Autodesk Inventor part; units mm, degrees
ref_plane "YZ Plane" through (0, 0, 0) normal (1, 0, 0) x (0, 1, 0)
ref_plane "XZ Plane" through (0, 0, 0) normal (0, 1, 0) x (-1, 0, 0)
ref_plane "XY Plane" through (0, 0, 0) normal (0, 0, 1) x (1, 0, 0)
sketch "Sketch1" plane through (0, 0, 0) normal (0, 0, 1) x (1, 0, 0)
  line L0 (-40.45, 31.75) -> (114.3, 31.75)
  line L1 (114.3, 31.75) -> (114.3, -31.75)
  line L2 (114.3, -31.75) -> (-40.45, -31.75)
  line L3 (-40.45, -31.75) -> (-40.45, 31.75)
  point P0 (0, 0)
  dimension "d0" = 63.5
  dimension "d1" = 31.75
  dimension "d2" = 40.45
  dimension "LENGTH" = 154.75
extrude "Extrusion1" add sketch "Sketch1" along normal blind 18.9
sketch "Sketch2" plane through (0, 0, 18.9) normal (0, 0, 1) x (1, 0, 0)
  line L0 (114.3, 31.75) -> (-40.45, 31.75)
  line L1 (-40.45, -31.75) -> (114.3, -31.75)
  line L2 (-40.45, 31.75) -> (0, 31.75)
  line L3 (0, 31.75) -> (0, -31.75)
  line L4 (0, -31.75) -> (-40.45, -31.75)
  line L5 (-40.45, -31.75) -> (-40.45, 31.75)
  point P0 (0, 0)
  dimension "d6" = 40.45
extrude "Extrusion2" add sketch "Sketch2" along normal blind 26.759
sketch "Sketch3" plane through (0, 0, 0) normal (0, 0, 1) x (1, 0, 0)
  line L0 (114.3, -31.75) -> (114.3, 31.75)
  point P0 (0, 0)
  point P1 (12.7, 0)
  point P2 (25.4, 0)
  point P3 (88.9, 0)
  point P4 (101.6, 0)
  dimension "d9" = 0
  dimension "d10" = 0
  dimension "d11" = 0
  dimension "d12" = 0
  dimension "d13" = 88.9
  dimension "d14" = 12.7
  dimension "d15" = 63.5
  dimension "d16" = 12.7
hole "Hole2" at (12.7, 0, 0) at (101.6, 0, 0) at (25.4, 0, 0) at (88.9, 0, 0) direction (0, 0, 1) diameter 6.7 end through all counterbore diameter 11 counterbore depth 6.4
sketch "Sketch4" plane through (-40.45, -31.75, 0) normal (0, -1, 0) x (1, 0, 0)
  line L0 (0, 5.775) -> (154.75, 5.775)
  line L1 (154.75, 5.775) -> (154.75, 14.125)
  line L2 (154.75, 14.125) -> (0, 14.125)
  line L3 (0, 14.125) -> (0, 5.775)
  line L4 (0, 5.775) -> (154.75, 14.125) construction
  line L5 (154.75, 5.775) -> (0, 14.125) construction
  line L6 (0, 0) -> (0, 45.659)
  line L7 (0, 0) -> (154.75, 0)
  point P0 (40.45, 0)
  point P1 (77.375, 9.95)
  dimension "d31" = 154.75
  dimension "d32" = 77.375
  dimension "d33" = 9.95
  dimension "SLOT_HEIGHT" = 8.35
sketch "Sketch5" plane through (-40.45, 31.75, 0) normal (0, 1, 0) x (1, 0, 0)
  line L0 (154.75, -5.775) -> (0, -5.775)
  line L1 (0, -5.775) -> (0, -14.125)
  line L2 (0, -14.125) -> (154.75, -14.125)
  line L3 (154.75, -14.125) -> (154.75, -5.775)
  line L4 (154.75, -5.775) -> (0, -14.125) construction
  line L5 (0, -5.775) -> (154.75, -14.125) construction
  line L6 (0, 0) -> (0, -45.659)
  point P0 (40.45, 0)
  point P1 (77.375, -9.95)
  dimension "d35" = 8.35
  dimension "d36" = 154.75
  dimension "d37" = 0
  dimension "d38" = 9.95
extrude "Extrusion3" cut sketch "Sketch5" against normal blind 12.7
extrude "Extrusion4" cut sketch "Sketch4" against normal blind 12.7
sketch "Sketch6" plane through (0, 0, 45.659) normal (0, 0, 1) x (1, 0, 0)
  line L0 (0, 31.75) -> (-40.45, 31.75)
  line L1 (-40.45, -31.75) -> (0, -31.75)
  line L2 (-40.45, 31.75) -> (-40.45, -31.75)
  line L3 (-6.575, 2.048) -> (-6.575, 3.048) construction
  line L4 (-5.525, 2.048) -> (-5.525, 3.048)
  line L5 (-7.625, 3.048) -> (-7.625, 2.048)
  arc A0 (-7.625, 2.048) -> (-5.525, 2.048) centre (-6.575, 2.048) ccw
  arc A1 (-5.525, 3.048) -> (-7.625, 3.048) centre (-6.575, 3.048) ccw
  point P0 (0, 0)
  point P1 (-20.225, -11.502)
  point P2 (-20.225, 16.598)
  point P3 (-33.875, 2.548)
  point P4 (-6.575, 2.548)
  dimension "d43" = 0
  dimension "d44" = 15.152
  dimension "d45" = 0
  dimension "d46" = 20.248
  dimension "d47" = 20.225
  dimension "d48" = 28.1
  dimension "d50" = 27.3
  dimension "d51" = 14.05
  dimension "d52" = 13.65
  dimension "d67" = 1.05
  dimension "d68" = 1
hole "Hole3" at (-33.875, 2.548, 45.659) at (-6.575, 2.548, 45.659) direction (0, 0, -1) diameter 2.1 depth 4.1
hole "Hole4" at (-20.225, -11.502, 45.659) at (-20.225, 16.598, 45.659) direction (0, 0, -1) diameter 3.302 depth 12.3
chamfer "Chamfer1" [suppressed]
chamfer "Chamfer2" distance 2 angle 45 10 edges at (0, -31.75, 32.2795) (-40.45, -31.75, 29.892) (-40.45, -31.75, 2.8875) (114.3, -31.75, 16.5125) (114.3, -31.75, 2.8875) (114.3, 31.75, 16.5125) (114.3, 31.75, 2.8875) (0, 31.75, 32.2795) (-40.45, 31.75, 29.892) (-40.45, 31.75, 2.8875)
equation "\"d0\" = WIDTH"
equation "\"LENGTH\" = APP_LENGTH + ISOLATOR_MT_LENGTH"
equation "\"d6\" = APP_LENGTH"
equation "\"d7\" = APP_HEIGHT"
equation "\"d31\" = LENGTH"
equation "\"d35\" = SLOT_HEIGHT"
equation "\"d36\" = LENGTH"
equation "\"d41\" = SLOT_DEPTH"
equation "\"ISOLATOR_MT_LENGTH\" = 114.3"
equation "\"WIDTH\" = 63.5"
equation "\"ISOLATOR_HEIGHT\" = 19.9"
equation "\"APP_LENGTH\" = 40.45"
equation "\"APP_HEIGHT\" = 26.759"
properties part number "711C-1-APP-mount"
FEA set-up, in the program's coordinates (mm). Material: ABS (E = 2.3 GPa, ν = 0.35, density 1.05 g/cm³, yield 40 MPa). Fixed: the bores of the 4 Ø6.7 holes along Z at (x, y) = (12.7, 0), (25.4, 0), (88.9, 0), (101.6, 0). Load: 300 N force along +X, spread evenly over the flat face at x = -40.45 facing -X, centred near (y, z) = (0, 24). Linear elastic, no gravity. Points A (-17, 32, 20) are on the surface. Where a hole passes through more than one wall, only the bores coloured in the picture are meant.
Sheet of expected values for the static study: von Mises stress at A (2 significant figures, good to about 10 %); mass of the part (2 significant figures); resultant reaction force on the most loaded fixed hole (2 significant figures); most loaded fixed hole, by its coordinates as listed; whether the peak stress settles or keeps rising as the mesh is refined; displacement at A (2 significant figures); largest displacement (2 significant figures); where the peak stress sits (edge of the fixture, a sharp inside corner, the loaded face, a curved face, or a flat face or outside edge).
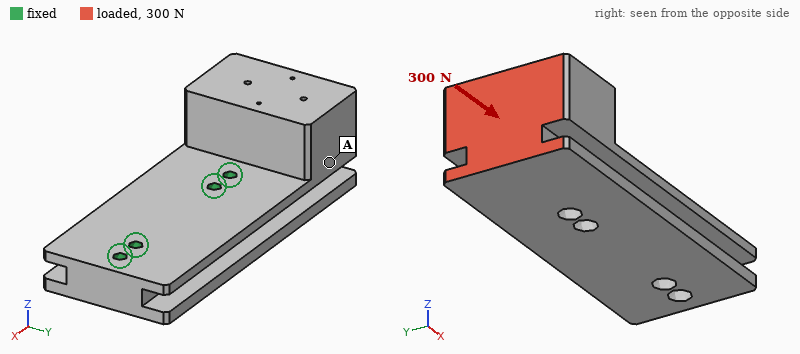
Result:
0.26 MPa
230 g
250 N
(12.7, 0)
keeps rising
0.047 mm
0.11 mm
edge of the fixture
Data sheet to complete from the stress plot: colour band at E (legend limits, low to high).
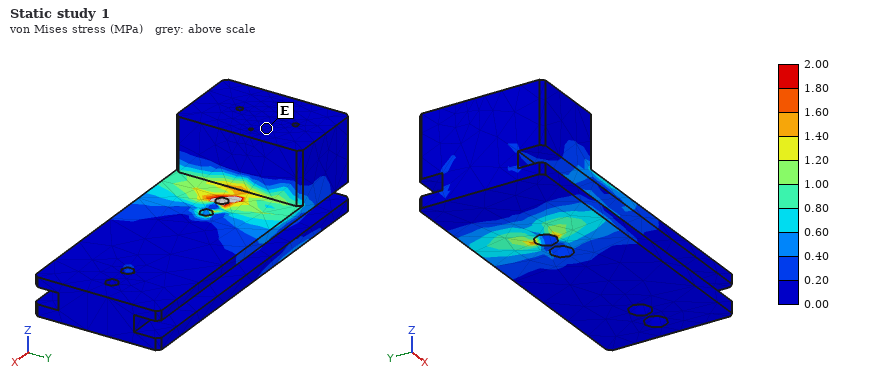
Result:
0.00 to 0.20 MPa
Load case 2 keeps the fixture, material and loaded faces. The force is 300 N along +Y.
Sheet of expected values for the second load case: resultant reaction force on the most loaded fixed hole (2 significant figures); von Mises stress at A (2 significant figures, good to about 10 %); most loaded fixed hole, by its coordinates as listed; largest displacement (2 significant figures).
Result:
560 N
0.39 MPa
(12.7, 0)
0.16 mm
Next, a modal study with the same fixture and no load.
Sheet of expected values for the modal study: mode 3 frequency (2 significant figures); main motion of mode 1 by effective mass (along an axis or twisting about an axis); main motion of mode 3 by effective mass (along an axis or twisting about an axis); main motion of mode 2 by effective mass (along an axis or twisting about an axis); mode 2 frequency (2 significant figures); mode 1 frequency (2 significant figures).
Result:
1300 Hz
along Z
along Y
along Y
780 Hz
610 Hz
